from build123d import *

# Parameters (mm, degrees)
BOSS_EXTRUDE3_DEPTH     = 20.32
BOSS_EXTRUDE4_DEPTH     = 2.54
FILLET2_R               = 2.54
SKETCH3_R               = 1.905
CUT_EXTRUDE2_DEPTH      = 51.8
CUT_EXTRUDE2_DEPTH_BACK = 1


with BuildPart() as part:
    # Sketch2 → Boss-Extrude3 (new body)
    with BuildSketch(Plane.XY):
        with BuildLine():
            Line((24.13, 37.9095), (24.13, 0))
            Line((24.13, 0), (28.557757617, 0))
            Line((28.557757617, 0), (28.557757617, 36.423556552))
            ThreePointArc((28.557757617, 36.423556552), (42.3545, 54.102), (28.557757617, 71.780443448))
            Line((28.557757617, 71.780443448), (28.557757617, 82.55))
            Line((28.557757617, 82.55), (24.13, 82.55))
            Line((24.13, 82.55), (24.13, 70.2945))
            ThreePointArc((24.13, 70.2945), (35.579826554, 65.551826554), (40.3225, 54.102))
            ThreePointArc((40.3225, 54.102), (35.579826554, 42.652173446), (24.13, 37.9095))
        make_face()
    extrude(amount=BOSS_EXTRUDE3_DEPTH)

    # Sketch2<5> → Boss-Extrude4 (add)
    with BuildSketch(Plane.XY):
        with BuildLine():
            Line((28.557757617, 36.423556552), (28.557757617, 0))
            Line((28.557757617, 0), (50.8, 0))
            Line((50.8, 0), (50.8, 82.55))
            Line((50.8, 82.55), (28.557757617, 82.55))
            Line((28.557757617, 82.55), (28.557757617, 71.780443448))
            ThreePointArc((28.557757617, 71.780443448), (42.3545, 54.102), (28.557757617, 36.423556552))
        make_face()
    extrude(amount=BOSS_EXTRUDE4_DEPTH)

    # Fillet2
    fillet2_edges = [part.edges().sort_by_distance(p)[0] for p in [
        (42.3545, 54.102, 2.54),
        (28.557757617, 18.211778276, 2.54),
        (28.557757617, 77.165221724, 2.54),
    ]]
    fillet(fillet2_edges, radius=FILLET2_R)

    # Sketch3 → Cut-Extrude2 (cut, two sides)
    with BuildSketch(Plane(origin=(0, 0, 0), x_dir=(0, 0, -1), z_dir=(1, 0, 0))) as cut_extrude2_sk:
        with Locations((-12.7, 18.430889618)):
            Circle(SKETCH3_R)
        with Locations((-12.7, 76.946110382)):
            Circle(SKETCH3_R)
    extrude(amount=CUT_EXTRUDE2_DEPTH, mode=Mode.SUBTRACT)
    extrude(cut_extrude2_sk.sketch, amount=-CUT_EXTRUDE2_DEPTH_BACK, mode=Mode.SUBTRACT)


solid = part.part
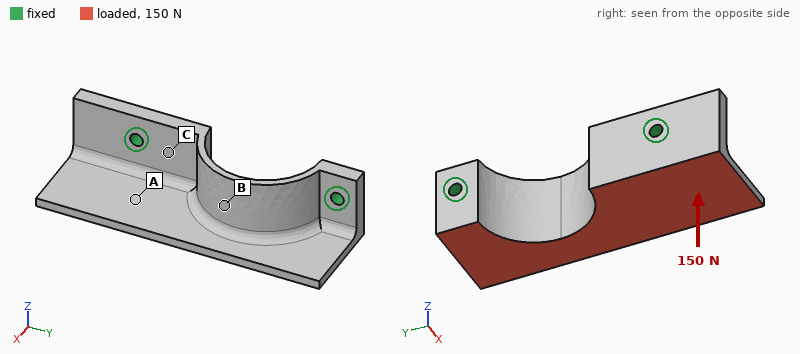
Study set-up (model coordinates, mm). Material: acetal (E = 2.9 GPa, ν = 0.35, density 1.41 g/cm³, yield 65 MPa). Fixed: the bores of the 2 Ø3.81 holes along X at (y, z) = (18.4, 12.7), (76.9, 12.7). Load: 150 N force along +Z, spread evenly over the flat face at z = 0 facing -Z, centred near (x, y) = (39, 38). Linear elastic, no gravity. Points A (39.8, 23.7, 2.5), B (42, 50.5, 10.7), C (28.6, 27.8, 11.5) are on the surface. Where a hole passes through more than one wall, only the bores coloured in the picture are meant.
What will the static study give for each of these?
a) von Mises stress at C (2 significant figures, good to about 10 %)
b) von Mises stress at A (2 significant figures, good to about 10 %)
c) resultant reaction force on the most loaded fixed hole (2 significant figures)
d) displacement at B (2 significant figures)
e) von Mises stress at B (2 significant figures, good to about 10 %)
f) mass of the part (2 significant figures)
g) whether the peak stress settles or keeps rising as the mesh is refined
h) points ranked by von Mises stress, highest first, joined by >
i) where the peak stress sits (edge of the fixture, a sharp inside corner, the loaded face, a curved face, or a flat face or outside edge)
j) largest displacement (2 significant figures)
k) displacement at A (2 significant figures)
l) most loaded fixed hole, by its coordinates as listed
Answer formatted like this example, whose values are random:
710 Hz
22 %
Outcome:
6.4 MPa
4.0 MPa
91 N
0.25 mm
1.9 MPa
14 g
keeps rising
C > A > B
edge of the fixture
0.92 mm
0.37 mm
(18.4, 12.7)
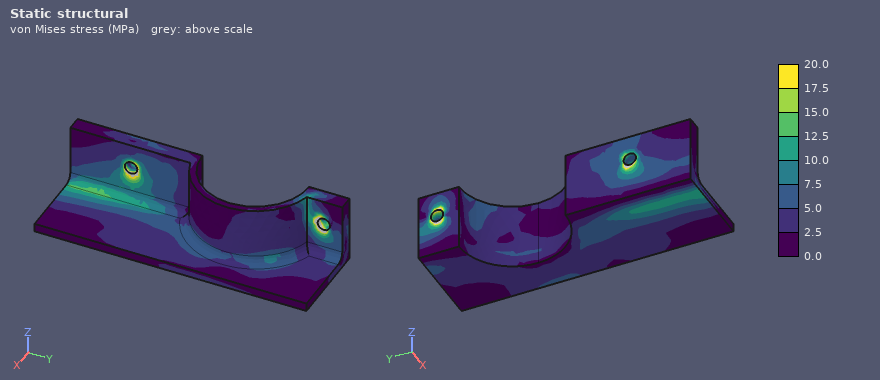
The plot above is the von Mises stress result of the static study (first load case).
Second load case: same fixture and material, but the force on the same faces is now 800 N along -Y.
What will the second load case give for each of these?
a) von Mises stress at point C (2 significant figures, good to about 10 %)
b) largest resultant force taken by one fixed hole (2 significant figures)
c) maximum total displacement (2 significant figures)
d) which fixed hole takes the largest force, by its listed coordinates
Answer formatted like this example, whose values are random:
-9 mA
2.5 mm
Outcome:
12 MPa
550 N
0.57 mm
(18.4, 12.7)
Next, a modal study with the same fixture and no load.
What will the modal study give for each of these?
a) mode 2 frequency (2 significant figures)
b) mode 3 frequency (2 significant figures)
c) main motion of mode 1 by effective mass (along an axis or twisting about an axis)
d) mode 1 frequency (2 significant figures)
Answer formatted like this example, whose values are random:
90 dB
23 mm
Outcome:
1300 Hz
1800 Hz
along Z
1000 Hz
